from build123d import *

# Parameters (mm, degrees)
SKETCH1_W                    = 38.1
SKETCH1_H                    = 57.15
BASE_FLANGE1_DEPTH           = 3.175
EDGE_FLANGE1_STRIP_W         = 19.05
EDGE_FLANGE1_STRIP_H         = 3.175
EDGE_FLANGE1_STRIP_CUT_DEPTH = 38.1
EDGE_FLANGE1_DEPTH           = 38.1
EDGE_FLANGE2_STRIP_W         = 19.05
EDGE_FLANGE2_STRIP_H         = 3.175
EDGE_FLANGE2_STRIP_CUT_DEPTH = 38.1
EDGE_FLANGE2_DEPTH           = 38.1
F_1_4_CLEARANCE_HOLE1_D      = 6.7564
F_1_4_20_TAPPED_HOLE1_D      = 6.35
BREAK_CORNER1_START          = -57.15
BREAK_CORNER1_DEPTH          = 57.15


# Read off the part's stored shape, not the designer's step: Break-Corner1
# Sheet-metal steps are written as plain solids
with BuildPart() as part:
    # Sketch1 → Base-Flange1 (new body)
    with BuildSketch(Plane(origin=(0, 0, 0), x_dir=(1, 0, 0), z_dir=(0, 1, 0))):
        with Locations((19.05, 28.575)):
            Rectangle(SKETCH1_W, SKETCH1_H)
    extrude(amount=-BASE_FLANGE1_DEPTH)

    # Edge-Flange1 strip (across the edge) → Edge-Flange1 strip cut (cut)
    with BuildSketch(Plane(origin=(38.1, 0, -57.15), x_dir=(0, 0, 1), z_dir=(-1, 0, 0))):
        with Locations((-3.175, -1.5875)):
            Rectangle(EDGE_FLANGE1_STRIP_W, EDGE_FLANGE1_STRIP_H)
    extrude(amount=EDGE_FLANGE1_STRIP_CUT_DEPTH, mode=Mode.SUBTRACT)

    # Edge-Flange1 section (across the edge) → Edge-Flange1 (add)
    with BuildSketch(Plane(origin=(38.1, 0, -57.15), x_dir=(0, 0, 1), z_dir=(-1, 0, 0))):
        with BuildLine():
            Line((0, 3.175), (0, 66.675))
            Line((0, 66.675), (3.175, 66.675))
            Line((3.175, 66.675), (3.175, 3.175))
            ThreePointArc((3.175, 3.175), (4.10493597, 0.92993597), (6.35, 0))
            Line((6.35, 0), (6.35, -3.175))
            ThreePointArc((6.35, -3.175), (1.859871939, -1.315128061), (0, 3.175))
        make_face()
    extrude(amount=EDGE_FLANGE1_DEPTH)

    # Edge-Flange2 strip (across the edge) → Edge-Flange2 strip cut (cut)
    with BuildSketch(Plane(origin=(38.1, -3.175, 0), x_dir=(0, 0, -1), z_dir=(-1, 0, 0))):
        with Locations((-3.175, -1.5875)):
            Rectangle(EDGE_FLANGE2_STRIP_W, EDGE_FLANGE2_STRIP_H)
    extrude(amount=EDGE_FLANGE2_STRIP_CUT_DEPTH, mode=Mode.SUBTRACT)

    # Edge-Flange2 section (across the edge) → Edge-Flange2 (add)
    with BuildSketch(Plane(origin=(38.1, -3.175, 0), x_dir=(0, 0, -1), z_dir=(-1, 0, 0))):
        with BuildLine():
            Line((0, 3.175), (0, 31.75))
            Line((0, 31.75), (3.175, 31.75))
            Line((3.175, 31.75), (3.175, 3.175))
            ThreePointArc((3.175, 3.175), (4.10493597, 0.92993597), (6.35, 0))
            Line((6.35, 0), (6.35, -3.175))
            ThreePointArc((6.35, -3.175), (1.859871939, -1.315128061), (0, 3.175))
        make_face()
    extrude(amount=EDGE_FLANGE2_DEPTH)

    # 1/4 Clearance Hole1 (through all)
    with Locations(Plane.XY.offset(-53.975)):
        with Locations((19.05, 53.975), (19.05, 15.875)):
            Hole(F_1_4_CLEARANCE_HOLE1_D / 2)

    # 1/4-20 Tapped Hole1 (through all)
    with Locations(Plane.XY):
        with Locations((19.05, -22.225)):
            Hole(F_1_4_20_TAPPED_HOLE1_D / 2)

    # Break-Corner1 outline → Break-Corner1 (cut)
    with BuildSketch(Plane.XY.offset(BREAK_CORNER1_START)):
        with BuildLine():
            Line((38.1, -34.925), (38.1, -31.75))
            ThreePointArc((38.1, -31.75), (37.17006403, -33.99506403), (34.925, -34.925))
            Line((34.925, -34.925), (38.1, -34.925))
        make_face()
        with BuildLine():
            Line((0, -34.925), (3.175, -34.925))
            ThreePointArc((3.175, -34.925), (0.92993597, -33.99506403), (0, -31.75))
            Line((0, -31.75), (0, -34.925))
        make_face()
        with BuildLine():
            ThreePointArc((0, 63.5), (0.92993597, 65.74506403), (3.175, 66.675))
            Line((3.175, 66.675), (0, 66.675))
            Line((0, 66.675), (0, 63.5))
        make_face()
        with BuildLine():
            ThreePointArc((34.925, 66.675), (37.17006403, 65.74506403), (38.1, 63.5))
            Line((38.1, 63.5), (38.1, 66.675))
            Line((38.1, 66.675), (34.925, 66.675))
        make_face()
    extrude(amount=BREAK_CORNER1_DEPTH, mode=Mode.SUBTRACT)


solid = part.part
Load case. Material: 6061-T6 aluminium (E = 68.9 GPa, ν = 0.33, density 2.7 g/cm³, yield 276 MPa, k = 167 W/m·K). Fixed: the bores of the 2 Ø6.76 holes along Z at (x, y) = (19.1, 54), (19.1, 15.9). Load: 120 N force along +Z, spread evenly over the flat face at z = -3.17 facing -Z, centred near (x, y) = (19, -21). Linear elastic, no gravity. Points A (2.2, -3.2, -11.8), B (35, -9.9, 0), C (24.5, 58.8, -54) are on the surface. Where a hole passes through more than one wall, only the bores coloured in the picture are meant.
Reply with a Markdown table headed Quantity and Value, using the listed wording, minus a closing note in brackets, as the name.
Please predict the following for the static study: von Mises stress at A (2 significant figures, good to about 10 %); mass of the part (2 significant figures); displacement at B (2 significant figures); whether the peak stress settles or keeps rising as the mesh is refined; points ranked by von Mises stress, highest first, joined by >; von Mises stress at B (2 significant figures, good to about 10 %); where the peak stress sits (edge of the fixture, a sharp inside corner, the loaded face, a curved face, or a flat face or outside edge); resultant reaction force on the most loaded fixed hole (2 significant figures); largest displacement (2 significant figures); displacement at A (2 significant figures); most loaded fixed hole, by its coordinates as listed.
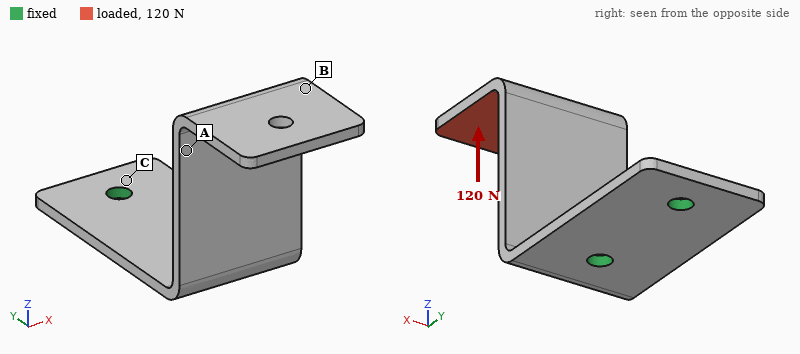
| Quantity | Value |
|---|---|
| von Mises stress at A | 35 MPa |
| mass of the part | 49 g |
| displacement at B | 0.91 mm |
| whether the peak stress settles or keeps rising as the mesh is refined | keeps rising |
| points ranked by von Mises stress, highest first, joined by > | A > B > C |
| von Mises stress at B | 19 MPa |
| where the peak stress sits | edge of the fixture |
| resultant reaction force on the most loaded fixed hole | 140 N |
| largest displacement | 1.3 mm |
| displacement at A | 0.61 mm |
| most loaded fixed hole, by its coordinates as listed | (19.1, 15.9) |
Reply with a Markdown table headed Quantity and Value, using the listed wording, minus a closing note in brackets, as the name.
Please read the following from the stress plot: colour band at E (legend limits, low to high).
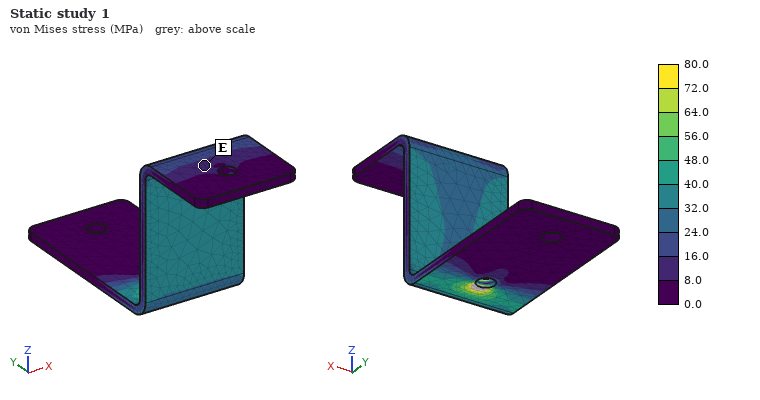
| Quantity | Value |
|---|---|
| colour band at E | 8.0 to 16.0 MPa |
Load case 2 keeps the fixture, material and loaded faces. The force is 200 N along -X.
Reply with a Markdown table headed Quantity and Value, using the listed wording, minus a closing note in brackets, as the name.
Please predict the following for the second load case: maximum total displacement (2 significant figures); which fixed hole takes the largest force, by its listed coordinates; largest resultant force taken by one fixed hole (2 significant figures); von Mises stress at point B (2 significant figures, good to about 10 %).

| Quantity | Value |
|---|---|
| maximum total displacement | 1.0 mm |
| which fixed hole takes the largest force, by its listed coordinates | (19.1, 15.9) |
| largest resultant force taken by one fixed hole | 340 N |
| von Mises stress at point B | 19 MPa |
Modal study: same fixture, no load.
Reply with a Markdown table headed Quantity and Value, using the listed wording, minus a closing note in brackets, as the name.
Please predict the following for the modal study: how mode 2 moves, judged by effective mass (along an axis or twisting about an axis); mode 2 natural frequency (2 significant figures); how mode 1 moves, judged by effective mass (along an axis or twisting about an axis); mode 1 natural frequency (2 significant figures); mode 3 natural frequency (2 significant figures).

| Quantity | Value |
|---|---|
| how mode 2 moves, judged by effective mass | along X |
| mode 2 natural frequency | 650 Hz |
| how mode 1 moves, judged by effective mass | along Y |
| mode 1 natural frequency | 330 Hz |
| mode 3 natural frequency | 1200 Hz |
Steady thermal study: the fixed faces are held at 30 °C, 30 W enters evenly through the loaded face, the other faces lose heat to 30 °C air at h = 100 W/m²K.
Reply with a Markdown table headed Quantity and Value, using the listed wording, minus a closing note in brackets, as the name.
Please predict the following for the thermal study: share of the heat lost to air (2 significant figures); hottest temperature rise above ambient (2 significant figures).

| Quantity | Value |
|---|---|
| share of the heat lost to air | 70 % |
| hottest temperature rise above ambient | 64 K |
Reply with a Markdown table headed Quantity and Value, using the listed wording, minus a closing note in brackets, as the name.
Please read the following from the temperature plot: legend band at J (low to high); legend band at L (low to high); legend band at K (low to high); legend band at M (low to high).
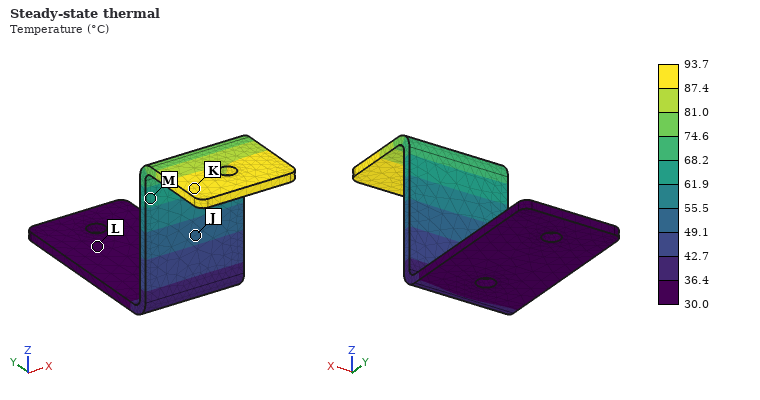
| Quantity | Value |
|---|---|
| legend band at J | 49.1 to 55.5 °C |
| legend band at L | 30.0 to 36.4 °C |
| legend band at K | 87.4 to 93.7 °C |
| legend band at M | 61.9 to 68.2 °C |
